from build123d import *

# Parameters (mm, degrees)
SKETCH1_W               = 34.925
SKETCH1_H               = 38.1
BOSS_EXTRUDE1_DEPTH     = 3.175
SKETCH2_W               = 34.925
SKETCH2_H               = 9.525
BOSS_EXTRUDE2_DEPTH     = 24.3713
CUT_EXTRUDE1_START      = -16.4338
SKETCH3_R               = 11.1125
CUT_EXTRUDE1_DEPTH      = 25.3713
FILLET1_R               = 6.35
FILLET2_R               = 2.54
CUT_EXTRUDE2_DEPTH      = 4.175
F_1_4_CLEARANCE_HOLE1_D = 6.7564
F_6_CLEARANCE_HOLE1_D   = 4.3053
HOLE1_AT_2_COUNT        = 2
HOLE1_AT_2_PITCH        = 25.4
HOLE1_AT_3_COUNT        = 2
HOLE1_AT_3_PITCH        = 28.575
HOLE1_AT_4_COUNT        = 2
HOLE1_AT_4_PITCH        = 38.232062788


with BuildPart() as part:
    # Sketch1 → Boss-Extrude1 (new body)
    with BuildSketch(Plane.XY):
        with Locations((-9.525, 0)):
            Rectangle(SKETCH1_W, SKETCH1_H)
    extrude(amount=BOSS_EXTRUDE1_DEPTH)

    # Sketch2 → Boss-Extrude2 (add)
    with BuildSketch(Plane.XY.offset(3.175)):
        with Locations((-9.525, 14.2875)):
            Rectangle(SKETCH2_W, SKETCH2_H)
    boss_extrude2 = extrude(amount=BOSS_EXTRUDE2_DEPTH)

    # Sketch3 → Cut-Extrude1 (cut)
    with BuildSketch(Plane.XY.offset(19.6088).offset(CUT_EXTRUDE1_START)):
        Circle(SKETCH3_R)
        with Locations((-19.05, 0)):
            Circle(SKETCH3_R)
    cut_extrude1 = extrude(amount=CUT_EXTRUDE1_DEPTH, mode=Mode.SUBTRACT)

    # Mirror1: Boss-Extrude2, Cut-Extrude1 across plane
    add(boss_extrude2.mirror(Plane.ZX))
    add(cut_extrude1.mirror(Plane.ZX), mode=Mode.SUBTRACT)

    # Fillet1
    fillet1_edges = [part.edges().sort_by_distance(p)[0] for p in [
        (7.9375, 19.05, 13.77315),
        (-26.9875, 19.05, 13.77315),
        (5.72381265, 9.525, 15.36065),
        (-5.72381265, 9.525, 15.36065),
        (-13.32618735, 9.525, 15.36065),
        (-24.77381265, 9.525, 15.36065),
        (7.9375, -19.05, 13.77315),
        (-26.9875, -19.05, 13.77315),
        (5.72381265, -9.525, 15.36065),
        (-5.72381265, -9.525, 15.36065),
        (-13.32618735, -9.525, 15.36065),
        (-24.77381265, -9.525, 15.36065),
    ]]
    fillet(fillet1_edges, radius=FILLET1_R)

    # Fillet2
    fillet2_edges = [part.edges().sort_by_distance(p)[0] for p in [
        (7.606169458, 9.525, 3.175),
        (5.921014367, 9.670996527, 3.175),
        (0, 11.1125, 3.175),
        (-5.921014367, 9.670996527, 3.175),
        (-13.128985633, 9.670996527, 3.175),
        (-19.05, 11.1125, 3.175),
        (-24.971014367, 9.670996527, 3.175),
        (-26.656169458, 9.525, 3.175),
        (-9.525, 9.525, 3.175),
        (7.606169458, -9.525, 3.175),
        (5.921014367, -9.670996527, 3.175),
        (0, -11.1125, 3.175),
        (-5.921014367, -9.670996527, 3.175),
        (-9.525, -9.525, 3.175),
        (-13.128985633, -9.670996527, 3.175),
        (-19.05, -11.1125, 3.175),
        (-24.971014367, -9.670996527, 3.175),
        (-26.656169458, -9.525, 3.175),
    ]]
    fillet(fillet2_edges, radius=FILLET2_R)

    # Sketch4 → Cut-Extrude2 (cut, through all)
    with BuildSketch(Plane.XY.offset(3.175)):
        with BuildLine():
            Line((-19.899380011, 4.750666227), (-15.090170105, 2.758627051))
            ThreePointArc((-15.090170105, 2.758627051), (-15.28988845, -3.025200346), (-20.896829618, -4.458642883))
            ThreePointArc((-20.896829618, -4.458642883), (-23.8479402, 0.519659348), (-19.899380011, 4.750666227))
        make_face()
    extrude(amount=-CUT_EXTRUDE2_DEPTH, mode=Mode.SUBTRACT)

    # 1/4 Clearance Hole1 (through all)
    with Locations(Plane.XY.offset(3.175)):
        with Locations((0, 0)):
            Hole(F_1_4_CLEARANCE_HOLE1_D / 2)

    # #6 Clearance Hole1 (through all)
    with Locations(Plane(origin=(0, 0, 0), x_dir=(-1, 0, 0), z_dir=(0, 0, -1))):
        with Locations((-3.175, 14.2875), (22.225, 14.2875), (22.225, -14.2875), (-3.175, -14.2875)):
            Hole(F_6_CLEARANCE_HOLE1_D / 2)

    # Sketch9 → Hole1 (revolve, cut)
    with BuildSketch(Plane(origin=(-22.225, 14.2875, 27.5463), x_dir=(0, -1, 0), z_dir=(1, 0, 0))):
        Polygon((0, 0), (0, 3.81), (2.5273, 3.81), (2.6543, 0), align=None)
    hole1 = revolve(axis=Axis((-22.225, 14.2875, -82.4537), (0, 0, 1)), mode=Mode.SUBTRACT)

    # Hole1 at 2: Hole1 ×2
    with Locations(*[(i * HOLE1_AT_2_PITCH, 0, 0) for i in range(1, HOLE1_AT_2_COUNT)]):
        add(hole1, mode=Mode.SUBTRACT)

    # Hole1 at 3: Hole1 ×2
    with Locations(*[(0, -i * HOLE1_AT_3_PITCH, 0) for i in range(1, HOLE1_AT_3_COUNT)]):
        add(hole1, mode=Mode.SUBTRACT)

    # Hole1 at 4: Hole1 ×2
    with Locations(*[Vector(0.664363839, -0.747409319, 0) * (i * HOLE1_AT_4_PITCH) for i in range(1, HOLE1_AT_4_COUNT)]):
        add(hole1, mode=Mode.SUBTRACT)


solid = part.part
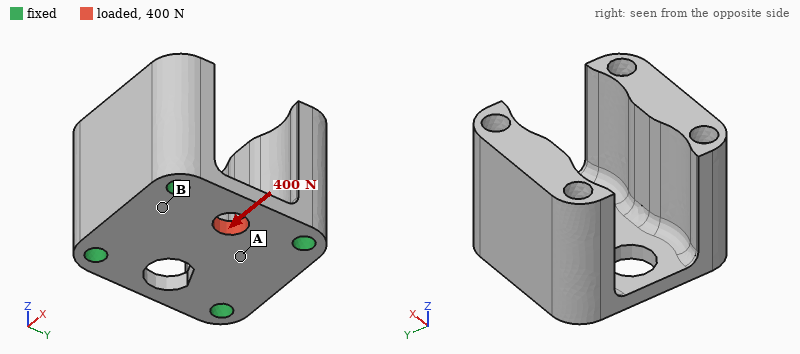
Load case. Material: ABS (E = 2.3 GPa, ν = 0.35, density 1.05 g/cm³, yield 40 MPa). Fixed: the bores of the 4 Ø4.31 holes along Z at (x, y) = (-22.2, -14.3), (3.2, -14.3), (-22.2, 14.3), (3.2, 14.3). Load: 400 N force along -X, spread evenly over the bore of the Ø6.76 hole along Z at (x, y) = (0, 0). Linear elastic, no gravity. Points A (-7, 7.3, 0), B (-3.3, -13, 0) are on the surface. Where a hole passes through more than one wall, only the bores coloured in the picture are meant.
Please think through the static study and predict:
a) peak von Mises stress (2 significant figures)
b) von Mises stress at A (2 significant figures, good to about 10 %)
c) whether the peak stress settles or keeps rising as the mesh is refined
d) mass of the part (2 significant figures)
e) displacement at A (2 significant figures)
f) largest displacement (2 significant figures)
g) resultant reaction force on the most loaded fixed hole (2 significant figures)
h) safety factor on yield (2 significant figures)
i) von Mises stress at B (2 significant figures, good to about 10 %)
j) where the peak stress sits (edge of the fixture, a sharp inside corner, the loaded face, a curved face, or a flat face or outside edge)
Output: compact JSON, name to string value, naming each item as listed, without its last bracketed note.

{"peak von Mises stress": "13 MPa", "von Mises stress at A": "4.3 MPa", "whether the peak stress settles or keeps rising as the mesh is refined": "settles", "mass of the part": "17 g", "displacement at A": "16 µm", "largest displacement": "63 µm", "resultant reaction force on the most loaded fixed hole": "120 N", "safety factor on yield": "3.0", "von Mises stress at B": "1.6 MPa", "where the peak stress sits": "the loaded face"}
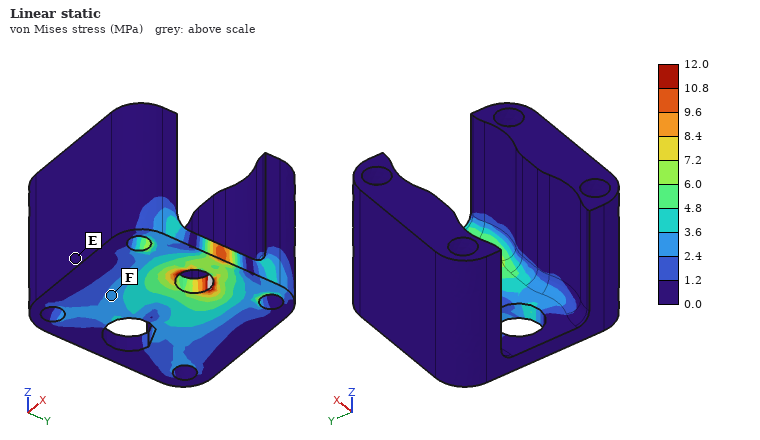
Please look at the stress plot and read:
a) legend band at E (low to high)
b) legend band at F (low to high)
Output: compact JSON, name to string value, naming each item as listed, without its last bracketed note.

{"legend band at E": "0.0 to 1.2 MPa", "legend band at F": "2.4 to 3.6 MPa"}
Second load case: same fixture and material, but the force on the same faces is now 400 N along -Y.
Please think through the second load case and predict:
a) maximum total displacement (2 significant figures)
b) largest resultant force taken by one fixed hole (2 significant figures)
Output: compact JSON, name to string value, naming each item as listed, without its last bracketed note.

{"maximum total displacement": "27 µm", "largest resultant force taken by one fixed hole": "160 N"}
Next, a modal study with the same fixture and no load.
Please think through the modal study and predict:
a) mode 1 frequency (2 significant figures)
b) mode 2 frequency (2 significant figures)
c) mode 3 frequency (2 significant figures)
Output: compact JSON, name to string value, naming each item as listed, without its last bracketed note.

{"mode 1 frequency": "9900 Hz", "mode 2 frequency": "11 kHz", "mode 3 frequency": "12 kHz"}
